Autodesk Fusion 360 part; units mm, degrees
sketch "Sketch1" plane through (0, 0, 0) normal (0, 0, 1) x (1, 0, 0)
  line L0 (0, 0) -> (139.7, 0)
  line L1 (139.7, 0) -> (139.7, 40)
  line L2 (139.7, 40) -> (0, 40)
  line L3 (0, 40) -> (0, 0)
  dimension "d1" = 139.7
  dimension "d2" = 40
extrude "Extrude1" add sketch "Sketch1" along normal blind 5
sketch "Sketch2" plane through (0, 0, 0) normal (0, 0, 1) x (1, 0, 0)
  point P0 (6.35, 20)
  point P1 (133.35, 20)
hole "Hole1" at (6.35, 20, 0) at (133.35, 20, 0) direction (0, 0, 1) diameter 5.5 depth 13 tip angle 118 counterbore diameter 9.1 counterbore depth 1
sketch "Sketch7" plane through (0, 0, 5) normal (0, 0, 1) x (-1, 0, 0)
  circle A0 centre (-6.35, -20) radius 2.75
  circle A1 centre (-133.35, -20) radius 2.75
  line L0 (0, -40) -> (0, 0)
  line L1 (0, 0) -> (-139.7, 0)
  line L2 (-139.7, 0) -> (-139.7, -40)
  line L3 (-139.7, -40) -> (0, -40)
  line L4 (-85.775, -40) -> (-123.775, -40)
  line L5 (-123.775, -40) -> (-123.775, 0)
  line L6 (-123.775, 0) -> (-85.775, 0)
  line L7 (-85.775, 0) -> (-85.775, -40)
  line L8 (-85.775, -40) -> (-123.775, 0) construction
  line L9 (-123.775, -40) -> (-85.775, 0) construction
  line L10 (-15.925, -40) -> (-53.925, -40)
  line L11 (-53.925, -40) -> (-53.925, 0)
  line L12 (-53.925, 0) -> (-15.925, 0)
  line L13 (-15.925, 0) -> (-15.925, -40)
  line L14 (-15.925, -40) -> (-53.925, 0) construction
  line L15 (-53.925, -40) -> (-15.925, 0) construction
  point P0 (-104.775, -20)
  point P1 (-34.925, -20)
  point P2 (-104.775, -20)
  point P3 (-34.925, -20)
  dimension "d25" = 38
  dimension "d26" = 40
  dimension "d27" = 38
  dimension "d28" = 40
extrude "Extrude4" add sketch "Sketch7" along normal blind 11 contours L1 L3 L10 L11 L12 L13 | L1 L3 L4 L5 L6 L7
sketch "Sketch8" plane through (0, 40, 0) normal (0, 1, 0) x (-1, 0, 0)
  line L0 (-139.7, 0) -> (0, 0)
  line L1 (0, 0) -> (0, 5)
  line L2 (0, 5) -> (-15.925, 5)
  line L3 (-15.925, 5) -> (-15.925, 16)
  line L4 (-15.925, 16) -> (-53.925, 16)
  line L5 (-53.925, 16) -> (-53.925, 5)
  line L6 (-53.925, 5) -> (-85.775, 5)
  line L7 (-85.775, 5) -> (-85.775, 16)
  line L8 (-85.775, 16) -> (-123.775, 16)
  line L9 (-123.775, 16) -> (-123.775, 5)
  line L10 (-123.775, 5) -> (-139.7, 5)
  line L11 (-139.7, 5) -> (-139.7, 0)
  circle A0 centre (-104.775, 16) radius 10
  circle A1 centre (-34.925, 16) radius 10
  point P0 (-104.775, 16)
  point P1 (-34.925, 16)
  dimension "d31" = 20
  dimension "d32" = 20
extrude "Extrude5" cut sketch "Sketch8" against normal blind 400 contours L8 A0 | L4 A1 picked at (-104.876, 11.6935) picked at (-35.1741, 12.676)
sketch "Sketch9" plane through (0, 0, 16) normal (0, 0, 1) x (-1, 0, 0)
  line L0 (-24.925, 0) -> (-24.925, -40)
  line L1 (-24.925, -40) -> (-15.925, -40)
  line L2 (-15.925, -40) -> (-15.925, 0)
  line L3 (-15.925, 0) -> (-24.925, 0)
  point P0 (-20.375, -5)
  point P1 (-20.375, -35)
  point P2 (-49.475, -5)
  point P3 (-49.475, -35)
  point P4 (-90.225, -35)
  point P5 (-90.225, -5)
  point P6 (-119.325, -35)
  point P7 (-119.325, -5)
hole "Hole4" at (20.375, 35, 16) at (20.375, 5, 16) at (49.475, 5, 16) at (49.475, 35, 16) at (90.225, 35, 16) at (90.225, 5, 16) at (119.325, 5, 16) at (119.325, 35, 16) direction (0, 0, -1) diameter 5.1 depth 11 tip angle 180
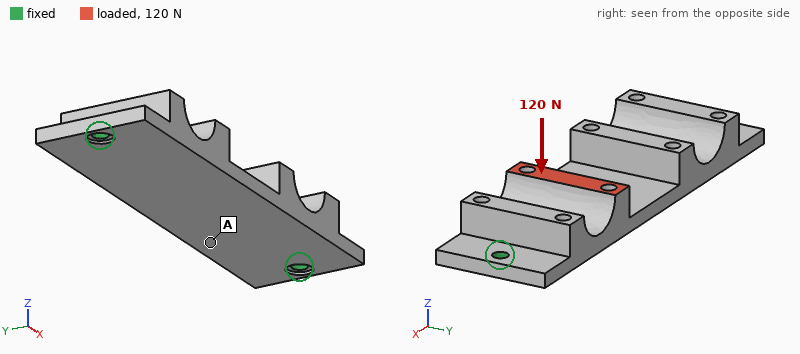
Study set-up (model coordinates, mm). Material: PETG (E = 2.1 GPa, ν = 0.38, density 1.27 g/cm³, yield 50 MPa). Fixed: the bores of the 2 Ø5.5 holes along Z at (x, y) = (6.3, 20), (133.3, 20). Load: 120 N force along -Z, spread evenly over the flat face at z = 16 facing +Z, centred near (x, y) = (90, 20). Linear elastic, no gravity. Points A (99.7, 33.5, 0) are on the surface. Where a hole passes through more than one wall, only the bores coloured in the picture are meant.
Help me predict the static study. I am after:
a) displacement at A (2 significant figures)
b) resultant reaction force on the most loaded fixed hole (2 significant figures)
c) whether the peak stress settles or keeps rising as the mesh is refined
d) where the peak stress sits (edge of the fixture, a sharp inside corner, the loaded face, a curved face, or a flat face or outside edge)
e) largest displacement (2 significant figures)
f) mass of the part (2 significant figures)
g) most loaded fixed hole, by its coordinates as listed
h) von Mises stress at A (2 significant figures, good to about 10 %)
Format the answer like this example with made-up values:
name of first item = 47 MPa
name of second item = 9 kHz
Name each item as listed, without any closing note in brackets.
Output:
displacement at A = 0.80 mm
resultant reaction force on the most loaded fixed hole = 85 N
whether the peak stress settles or keeps rising as the mesh is refined = keeps rising
where the peak stress sits = edge of the fixture
largest displacement = 1.2 mm
mass of the part = 59 g
most loaded fixed hole, by its coordinates as listed = (133.3, 20)
von Mises stress at A = 2.8 MPa
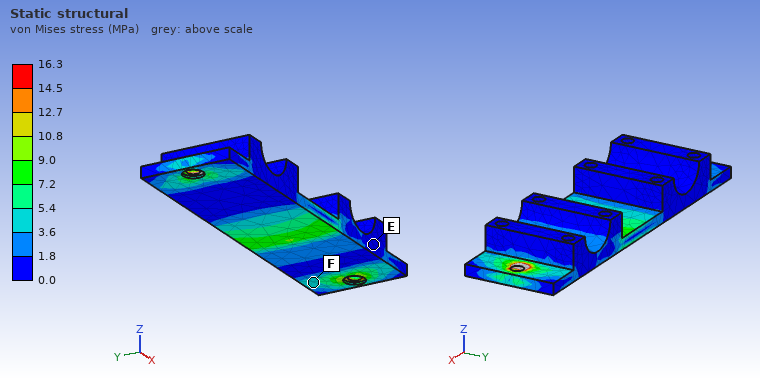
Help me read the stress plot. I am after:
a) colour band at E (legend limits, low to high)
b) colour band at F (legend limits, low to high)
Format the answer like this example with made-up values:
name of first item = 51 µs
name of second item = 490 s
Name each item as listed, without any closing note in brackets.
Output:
colour band at E = 0.0 to 1.8 MPa
colour band at F = 3.6 to 5.4 MPa
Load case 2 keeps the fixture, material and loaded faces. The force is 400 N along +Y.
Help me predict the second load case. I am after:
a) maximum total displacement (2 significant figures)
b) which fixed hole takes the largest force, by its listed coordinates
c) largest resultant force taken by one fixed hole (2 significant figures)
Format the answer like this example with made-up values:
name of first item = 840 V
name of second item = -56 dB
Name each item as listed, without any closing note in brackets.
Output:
maximum total displacement = 1.5 mm
which fixed hole takes the largest force, by its listed coordinates = (133.3, 20)
largest resultant force taken by one fixed hole = 270 N
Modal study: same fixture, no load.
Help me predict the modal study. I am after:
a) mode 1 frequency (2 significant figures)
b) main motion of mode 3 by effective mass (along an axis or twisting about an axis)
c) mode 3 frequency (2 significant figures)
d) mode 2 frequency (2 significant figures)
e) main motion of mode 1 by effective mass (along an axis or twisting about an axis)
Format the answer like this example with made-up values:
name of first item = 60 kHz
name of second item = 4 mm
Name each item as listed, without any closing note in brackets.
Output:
mode 1 frequency = 310 Hz
main motion of mode 3 by effective mass = twisting about Y
mode 3 frequency = 980 Hz
mode 2 frequency = 660 Hz
main motion of mode 1 by effective mass = along Z
